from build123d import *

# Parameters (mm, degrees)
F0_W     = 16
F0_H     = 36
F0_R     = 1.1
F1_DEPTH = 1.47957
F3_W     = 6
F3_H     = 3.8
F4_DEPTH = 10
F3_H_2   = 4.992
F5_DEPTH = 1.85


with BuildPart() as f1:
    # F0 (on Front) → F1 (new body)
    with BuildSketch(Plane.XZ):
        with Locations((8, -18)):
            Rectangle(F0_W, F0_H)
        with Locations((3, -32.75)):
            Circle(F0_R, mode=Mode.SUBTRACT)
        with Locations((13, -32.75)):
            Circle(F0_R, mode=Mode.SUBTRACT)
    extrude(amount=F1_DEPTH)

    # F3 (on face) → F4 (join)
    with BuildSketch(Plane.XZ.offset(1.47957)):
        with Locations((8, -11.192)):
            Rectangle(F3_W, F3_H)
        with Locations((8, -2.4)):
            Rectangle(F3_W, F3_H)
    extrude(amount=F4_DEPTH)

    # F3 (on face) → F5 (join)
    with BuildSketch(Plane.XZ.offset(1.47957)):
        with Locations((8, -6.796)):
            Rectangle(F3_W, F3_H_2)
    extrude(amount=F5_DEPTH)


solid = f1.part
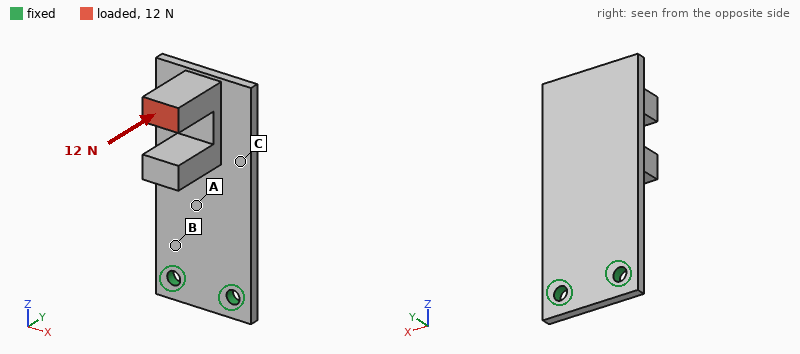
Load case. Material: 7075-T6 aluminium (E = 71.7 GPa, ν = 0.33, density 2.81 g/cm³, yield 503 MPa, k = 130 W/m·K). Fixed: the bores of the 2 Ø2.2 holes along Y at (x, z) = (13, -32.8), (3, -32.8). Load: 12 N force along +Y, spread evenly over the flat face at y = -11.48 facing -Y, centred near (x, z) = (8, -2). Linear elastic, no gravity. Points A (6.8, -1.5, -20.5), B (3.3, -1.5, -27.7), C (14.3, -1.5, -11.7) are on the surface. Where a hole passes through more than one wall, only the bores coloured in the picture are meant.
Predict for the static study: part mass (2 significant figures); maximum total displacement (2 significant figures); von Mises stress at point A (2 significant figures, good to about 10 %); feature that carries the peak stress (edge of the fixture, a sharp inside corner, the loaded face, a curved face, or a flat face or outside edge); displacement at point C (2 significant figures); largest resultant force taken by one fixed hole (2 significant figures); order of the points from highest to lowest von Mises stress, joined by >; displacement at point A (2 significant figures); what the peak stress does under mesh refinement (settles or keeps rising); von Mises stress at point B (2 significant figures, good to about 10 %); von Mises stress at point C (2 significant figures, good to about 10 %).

3.8 g
0.39 mm
35 MPa
edge of the fixture
0.18 mm
6.0 N
B > A > C
0.071 mm
keeps rising
48 MPa
11 MPa
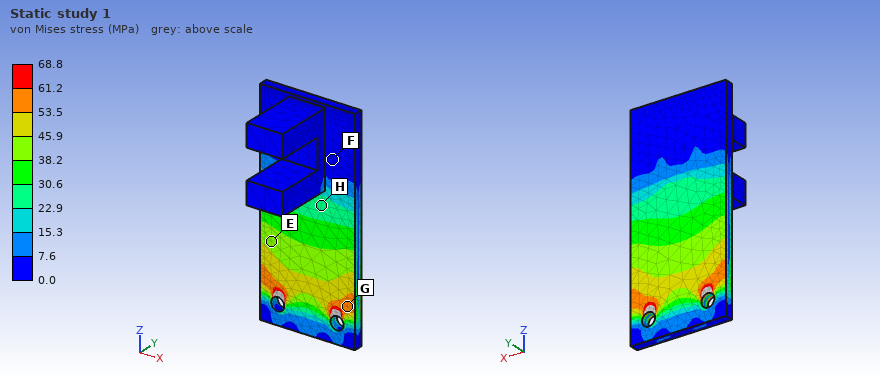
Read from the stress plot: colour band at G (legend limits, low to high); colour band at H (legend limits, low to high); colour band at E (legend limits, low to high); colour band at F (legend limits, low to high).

53.5 to 61.2 MPa
22.9 to 30.6 MPa
38.2 to 45.9 MPa
0.0 to 7.6 MPa
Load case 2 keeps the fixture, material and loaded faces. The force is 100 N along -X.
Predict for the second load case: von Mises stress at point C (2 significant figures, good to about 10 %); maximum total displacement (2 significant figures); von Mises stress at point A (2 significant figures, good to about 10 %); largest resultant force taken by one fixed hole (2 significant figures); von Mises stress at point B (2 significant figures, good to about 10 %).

110 MPa
0.49 mm
160 MPa
290 N
120 MPa
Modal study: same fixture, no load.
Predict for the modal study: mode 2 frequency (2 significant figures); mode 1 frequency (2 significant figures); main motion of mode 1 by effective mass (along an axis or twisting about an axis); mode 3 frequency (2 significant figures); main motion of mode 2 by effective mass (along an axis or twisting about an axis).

2900 Hz
730 Hz
along Y
4900 Hz
along X
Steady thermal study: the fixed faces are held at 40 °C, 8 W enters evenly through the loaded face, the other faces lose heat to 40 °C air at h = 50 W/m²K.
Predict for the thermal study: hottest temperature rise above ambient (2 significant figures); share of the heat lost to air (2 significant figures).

76 K
33 %
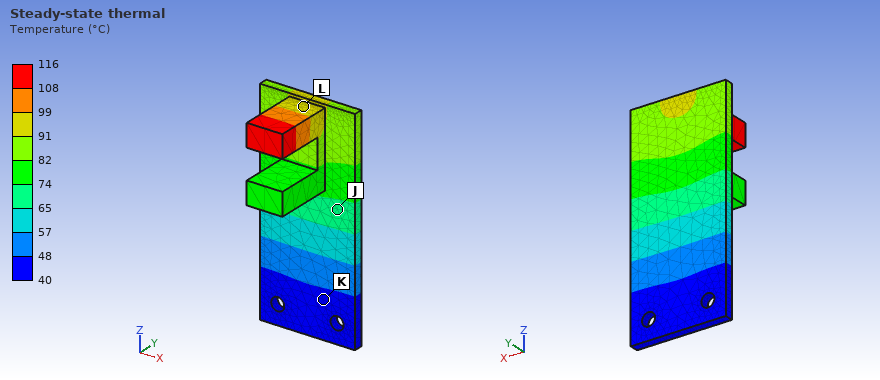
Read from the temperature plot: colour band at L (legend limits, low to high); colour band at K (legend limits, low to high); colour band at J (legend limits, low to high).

91 to 99 °C
40 to 48 °C
65 to 74 °C
